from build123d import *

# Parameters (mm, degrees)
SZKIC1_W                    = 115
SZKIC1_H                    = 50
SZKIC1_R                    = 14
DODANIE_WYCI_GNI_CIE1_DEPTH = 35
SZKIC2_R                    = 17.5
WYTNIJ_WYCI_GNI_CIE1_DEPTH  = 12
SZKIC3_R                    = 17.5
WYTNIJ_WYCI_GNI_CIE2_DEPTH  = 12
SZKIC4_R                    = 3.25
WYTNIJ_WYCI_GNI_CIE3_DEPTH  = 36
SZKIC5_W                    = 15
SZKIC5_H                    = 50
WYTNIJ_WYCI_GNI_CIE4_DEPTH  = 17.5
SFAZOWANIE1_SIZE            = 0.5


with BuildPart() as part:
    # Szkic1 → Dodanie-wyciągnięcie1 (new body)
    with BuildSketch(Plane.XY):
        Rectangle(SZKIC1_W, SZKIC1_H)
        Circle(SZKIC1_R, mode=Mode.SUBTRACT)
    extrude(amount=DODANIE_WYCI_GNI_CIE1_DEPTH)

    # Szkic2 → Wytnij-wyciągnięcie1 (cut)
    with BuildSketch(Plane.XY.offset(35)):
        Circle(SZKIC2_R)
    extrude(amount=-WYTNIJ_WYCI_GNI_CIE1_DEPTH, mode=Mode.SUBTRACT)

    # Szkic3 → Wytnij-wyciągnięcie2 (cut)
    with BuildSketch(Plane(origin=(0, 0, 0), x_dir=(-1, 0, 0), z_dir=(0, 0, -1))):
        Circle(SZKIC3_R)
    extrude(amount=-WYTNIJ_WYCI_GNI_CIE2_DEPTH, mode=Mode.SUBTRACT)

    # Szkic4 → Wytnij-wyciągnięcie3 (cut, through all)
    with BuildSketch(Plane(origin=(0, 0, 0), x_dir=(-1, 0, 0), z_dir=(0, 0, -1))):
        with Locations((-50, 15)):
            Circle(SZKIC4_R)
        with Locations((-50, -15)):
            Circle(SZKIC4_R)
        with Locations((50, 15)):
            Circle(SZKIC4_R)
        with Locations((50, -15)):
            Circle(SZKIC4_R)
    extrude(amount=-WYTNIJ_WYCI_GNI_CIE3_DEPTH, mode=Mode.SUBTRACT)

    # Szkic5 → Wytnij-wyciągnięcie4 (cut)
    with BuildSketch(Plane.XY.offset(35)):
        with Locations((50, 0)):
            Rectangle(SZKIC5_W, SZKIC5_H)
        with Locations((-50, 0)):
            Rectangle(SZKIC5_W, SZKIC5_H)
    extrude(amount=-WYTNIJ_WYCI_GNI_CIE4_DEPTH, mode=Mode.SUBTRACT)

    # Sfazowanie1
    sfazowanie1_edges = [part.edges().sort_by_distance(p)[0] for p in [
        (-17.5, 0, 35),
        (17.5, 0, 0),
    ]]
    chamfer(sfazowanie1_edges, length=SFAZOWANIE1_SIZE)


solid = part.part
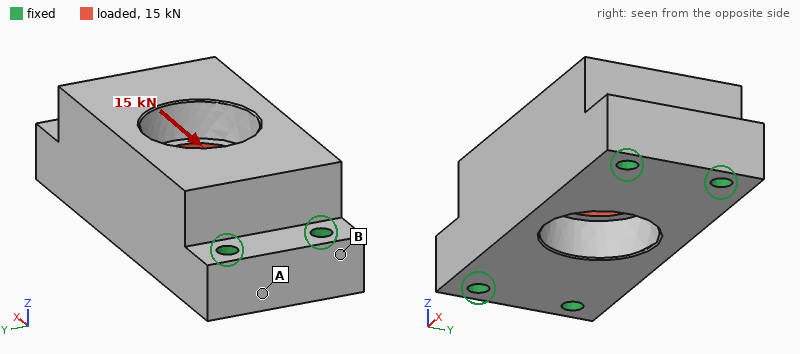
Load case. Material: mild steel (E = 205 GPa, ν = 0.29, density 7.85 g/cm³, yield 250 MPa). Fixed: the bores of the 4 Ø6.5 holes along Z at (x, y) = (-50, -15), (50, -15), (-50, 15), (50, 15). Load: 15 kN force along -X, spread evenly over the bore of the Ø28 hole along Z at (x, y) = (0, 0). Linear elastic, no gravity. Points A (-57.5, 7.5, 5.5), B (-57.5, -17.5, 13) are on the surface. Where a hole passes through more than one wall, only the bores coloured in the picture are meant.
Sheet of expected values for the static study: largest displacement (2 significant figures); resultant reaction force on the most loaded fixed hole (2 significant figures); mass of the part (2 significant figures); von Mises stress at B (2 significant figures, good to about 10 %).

2.5 µm
3.8 kN
1.1 kg
5.6 MPa
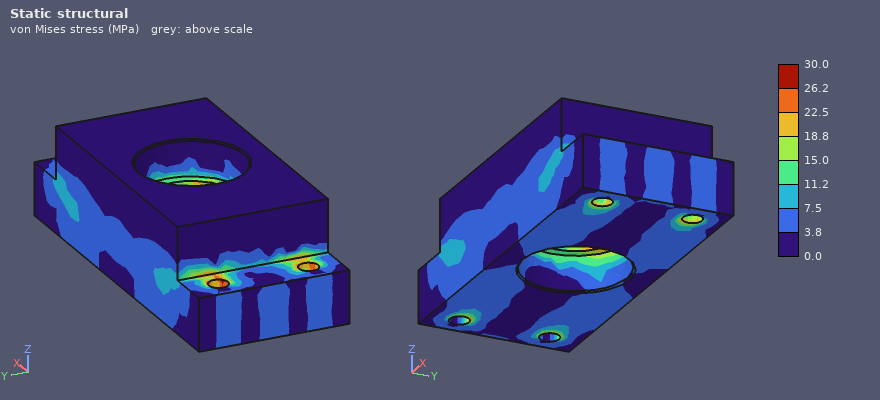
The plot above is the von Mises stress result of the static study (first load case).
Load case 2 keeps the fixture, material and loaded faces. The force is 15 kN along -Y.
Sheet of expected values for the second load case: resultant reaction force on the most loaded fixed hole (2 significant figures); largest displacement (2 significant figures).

5.7 kN
7.5 µm
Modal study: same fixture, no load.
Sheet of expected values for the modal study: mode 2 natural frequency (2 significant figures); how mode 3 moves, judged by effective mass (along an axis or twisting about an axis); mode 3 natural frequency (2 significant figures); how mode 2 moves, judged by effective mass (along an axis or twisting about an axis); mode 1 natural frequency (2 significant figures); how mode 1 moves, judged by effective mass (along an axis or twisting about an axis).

9300 Hz
along Y
13 kHz
along Y
8400 Hz
along Z
